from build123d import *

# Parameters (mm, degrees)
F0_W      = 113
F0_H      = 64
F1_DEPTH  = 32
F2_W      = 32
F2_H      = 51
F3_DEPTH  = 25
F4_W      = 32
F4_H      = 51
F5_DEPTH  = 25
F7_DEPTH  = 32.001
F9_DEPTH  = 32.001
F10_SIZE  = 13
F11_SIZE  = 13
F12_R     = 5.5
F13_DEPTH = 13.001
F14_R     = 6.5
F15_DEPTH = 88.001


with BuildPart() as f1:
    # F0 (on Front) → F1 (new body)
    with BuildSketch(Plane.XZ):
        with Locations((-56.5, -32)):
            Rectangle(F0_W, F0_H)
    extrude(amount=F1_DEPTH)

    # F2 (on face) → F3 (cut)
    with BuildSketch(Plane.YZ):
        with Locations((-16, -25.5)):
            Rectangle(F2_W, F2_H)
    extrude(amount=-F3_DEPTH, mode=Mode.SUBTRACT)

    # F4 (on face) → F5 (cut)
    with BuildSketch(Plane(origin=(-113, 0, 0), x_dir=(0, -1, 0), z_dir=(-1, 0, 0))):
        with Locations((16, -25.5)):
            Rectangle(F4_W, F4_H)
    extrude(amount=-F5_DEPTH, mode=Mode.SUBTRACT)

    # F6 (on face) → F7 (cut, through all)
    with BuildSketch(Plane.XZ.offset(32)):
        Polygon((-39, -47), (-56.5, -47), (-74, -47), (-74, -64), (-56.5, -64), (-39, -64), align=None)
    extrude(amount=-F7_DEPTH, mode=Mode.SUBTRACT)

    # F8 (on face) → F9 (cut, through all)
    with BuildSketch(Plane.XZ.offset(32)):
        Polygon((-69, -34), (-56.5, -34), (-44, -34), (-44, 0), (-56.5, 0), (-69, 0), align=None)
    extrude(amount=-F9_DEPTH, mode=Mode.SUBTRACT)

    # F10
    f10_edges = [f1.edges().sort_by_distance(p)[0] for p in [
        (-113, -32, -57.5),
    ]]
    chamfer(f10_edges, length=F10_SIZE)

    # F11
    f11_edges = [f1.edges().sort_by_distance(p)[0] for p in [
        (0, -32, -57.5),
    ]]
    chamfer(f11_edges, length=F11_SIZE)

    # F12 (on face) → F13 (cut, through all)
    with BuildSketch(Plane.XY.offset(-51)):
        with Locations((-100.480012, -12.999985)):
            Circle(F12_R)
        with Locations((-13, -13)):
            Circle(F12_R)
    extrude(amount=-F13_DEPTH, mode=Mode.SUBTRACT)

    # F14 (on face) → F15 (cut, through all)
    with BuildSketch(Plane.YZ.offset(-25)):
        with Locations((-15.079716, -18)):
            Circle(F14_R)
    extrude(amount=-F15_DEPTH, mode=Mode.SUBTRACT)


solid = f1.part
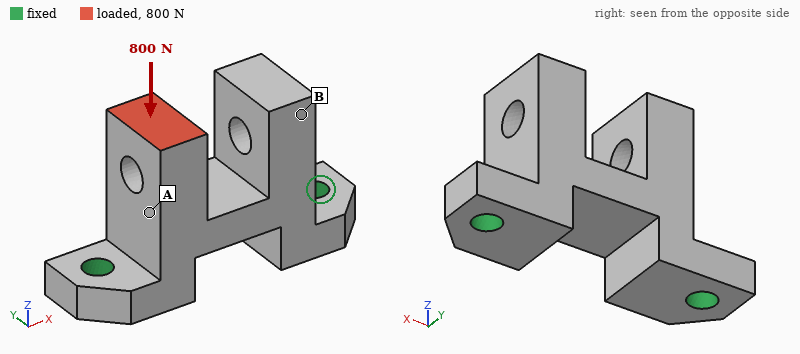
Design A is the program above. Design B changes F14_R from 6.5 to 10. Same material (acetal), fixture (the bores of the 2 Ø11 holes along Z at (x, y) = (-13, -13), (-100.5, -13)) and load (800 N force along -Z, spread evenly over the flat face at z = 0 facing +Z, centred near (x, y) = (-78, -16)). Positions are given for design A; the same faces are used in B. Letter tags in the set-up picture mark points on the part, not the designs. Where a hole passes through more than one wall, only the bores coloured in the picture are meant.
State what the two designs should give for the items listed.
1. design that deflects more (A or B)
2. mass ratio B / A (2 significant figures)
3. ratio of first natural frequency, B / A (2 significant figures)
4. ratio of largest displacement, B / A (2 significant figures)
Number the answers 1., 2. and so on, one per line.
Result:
1. B
2. 0.93
3. 1.1
4. 1.3
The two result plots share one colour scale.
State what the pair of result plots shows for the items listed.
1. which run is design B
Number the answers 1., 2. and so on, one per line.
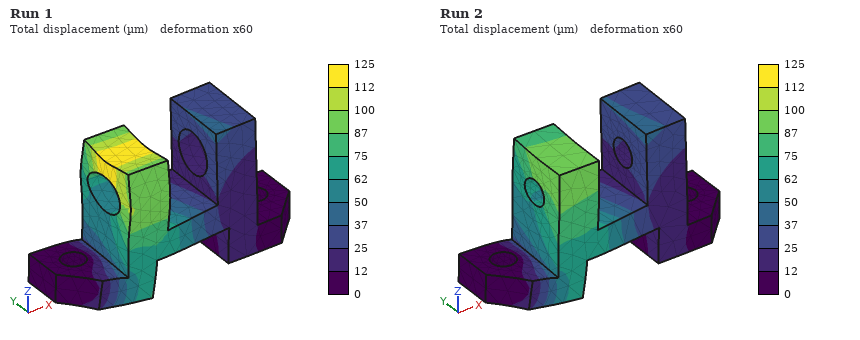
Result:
1. Run 1
